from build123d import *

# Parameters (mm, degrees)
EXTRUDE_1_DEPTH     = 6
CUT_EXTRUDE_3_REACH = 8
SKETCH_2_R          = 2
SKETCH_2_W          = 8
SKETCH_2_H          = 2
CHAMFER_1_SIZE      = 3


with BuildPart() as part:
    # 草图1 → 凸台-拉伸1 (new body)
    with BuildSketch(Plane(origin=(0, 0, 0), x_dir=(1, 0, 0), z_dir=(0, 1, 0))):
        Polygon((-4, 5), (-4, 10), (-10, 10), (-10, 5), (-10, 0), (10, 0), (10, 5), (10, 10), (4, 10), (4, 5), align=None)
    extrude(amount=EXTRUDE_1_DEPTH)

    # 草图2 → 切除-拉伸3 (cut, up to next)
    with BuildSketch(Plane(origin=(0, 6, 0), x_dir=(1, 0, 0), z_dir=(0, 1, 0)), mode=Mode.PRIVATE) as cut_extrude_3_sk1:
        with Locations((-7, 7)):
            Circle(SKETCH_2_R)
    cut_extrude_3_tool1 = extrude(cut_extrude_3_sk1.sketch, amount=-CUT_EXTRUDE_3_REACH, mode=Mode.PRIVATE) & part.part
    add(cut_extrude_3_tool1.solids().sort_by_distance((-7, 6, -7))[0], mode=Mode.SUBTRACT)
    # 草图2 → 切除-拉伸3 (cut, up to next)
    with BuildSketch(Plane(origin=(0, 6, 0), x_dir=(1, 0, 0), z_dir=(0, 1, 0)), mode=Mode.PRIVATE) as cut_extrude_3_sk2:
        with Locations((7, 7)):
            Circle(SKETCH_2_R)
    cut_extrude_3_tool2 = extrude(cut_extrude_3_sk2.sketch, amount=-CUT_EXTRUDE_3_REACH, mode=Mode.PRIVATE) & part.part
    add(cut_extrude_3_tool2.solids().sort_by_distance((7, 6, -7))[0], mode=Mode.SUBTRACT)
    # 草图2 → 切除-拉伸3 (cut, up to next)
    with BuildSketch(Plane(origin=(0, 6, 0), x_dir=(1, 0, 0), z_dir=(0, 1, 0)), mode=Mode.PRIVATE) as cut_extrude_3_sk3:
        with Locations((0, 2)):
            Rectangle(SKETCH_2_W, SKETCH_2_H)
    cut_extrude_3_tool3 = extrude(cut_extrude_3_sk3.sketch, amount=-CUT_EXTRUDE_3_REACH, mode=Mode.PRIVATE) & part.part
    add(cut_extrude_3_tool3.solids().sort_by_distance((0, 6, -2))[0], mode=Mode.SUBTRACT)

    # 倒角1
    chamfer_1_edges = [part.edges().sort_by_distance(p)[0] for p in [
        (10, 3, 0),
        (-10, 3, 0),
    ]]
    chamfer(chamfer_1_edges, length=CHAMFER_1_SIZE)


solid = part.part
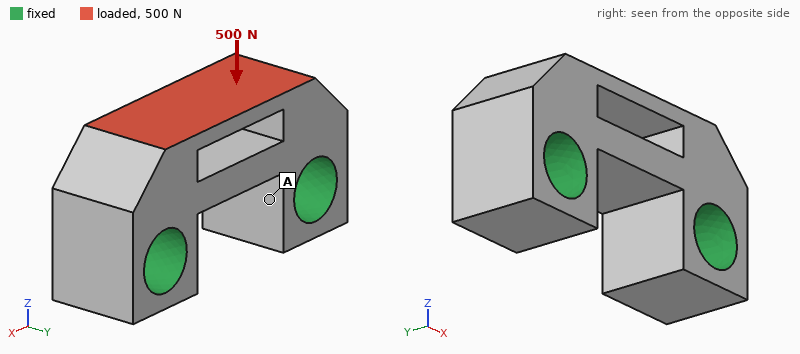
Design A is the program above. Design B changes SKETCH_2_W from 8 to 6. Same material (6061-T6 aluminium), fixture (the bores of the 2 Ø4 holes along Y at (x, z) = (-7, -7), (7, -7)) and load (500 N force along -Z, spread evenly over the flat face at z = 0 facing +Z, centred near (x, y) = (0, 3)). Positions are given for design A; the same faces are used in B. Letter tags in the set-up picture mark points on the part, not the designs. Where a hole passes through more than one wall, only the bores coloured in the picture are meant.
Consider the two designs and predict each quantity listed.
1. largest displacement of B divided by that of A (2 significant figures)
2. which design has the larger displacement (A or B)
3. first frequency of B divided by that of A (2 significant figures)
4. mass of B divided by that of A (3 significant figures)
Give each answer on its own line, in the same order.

0.43
A
1.3
1.04
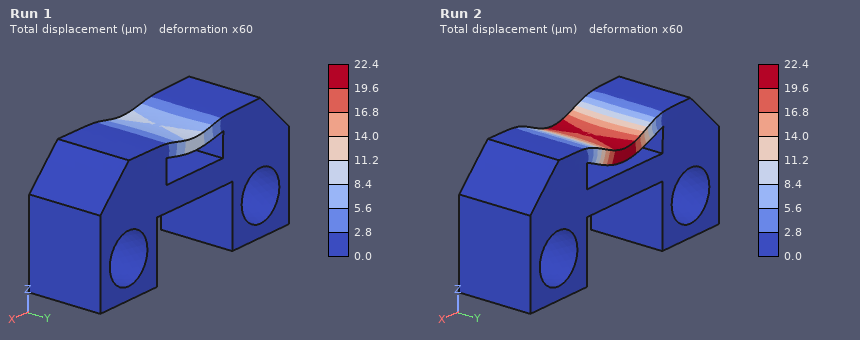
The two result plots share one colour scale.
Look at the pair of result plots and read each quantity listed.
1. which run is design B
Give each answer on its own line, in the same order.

Run 1
